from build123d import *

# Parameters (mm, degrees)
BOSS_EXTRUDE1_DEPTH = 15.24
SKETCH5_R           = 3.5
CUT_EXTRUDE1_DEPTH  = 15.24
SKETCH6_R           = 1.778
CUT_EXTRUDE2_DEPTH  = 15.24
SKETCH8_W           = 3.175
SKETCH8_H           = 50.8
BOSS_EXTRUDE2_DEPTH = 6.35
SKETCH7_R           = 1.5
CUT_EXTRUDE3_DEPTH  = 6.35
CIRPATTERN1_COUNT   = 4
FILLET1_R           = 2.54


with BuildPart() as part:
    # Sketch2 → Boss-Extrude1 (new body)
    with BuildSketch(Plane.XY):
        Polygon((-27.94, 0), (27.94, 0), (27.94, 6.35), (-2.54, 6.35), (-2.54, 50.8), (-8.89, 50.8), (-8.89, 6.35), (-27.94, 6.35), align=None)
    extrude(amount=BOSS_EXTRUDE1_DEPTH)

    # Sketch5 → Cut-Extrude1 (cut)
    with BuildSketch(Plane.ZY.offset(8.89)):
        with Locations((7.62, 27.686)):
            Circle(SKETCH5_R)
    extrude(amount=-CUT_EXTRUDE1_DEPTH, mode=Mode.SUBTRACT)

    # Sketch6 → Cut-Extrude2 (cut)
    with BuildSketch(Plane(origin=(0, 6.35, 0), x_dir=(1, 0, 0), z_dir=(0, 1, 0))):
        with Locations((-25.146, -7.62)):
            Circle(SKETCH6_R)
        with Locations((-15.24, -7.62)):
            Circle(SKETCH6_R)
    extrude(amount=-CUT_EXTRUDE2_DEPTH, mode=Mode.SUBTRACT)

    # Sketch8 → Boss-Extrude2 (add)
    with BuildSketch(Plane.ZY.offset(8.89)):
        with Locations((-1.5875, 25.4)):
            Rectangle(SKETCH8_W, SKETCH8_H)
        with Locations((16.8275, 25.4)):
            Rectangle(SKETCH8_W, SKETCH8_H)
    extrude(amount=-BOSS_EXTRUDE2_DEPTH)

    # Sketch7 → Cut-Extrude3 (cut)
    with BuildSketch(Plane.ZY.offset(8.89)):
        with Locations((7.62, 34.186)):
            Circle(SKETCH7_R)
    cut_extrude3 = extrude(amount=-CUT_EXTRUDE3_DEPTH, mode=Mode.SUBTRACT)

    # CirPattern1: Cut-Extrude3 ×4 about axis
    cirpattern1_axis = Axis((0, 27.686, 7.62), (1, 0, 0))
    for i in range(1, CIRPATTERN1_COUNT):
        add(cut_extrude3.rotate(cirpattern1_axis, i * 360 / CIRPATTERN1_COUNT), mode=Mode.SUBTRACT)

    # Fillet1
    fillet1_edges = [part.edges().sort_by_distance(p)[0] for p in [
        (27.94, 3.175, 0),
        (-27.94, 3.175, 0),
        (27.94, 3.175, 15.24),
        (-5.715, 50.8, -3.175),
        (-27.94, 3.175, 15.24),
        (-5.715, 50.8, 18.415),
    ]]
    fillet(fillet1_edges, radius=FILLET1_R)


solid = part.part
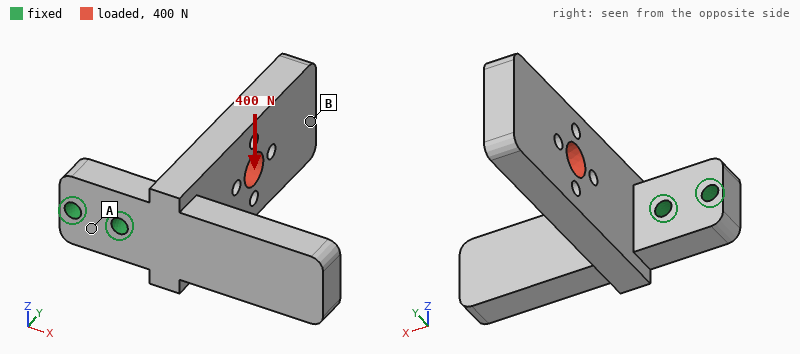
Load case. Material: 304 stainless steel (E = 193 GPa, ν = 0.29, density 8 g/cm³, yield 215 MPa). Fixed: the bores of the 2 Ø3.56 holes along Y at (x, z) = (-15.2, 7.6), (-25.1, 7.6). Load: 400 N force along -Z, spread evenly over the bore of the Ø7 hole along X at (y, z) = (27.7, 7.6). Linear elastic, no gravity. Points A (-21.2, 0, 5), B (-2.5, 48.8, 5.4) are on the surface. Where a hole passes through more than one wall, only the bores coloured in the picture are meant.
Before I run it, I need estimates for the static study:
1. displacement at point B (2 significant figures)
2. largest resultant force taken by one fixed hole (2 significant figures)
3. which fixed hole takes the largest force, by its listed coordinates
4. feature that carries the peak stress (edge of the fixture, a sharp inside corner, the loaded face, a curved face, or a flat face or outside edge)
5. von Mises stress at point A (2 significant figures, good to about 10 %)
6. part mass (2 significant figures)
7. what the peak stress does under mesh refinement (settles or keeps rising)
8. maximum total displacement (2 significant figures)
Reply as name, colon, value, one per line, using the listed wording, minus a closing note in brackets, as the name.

displacement at point B: 50 µm
largest resultant force taken by one fixed hole: 620 N
which fixed hole takes the largest force, by its listed coordinates: (-15.2, 7.6)
feature that carries the peak stress: edge of the fixture
von Mises stress at point A: 23 MPa
part mass: 89 g
what the peak stress does under mesh refinement: keeps rising
maximum total displacement: 53 µm
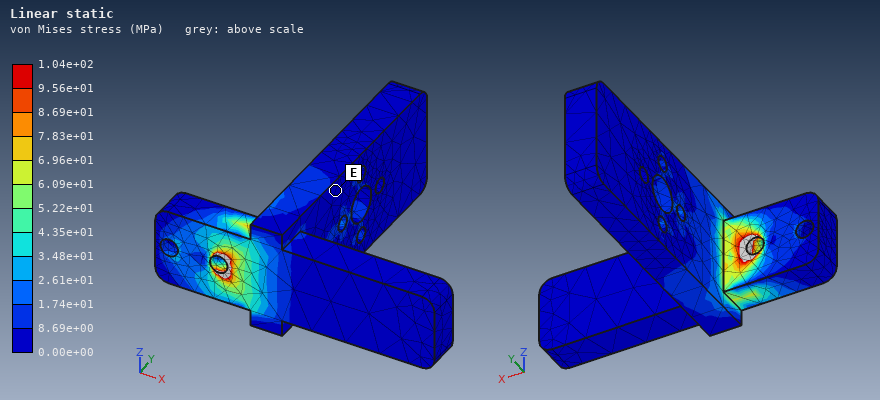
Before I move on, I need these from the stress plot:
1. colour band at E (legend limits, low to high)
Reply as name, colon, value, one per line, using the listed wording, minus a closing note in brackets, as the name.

colour band at E: 0.00e+00 to 8.69e+00 MPa
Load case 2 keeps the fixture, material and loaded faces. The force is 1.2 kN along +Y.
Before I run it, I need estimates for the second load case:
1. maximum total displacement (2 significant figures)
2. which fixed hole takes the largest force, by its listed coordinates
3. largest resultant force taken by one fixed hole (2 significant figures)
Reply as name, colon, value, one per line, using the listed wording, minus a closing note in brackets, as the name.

maximum total displacement: 45 µm
which fixed hole takes the largest force, by its listed coordinates: (-15.2, 7.6)
largest resultant force taken by one fixed hole: 1.4 kN
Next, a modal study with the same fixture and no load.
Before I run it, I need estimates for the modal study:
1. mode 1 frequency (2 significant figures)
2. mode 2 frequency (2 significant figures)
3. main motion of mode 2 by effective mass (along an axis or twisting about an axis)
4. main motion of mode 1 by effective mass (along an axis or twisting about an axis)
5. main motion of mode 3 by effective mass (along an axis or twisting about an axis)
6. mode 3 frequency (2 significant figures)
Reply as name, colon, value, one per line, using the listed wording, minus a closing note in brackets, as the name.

mode 1 frequency: 1500 Hz
mode 2 frequency: 2400 Hz
main motion of mode 2 by effective mass: along Z
main motion of mode 1 by effective mass: along X
main motion of mode 3 by effective mass: along Y
mode 3 frequency: 3600 Hz
